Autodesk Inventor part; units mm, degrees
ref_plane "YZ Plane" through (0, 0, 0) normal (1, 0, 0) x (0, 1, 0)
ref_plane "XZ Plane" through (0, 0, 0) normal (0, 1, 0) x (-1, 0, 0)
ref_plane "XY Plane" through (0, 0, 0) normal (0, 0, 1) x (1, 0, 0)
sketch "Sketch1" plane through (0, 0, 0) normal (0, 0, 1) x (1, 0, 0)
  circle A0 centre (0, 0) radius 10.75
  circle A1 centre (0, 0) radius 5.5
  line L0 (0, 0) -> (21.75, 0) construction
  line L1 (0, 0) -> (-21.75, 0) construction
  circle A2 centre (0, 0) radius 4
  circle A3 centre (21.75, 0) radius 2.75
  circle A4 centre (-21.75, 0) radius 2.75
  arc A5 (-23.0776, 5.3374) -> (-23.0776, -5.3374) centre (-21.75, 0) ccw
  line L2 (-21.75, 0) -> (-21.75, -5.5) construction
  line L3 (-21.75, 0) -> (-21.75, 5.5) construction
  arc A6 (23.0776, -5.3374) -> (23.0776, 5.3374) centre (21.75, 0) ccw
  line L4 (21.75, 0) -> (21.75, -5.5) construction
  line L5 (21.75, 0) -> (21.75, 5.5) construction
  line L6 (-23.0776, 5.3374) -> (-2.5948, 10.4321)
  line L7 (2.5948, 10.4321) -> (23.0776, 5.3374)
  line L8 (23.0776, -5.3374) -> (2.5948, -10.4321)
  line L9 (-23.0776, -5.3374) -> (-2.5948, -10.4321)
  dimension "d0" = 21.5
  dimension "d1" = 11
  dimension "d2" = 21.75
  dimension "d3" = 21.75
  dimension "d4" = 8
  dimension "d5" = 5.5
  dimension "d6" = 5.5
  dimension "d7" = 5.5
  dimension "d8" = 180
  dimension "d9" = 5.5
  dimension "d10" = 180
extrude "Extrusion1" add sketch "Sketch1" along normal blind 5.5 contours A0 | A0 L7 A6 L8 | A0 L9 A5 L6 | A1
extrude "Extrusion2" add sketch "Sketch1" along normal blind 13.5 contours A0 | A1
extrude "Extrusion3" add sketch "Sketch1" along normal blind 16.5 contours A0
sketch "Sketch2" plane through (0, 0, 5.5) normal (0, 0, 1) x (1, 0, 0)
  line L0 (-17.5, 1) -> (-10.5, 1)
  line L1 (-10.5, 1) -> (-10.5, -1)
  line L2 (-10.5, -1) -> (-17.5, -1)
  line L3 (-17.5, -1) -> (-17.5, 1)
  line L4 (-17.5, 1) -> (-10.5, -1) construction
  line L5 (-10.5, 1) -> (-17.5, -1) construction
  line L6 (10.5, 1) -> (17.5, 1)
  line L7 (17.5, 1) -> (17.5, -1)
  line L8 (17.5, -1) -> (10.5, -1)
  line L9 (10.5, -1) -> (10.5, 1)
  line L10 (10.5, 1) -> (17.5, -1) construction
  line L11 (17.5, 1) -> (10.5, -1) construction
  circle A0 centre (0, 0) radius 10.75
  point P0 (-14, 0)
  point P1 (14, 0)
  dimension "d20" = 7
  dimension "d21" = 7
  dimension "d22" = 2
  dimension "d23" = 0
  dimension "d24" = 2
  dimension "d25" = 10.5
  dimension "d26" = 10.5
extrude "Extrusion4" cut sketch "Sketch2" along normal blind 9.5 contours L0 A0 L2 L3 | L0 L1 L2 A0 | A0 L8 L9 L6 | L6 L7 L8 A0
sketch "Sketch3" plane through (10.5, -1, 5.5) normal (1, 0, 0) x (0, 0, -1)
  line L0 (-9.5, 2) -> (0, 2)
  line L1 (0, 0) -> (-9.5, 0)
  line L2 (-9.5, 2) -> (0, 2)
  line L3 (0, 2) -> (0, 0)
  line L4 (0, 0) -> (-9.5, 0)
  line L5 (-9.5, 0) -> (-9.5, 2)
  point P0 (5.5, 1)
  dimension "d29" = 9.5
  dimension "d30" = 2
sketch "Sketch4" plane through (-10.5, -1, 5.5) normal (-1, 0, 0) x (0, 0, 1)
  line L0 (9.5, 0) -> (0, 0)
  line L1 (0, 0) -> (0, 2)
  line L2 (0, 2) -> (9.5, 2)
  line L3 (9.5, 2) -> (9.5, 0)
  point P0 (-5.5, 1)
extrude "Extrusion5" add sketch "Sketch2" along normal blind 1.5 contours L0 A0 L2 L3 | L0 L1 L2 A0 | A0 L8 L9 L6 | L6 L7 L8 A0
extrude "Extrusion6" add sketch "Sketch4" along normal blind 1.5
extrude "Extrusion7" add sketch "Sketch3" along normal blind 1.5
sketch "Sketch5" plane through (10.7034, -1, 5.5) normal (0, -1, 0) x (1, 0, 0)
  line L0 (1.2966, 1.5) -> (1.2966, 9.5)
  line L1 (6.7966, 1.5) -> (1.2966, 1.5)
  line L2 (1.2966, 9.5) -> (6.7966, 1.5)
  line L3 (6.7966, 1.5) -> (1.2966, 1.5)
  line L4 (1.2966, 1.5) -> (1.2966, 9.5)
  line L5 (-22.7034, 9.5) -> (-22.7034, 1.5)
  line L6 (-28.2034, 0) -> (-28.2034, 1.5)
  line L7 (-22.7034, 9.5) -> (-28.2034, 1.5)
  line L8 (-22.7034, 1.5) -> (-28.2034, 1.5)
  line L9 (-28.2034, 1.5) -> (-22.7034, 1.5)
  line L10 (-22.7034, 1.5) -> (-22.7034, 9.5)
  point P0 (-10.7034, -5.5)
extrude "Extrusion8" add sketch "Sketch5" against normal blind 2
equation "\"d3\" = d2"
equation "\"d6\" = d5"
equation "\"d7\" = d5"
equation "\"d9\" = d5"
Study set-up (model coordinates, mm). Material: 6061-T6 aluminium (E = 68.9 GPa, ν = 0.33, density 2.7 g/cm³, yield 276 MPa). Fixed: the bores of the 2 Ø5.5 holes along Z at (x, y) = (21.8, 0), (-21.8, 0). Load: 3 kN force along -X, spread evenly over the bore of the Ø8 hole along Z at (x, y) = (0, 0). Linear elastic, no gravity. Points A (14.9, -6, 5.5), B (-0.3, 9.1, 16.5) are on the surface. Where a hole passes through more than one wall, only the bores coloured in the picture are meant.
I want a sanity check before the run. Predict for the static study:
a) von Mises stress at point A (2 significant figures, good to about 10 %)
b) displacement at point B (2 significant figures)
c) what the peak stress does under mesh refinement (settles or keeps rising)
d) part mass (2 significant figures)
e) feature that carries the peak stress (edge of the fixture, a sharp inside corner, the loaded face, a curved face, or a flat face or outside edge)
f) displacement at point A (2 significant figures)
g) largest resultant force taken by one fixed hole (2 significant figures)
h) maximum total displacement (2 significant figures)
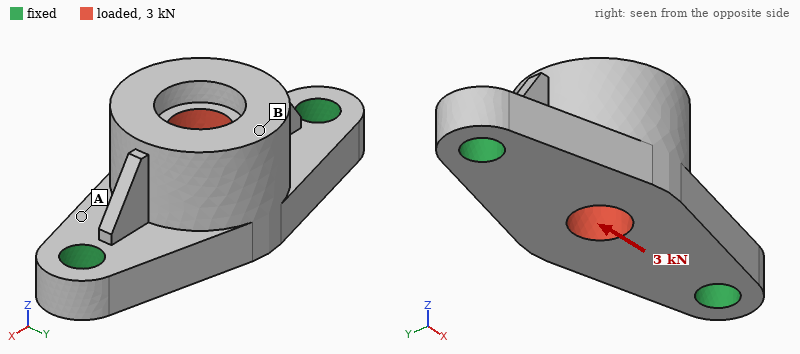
18 MPa
6.5 µm
keeps rising
20 g
a sharp inside corner
2.3 µm
1.5 kN
6.8 µm
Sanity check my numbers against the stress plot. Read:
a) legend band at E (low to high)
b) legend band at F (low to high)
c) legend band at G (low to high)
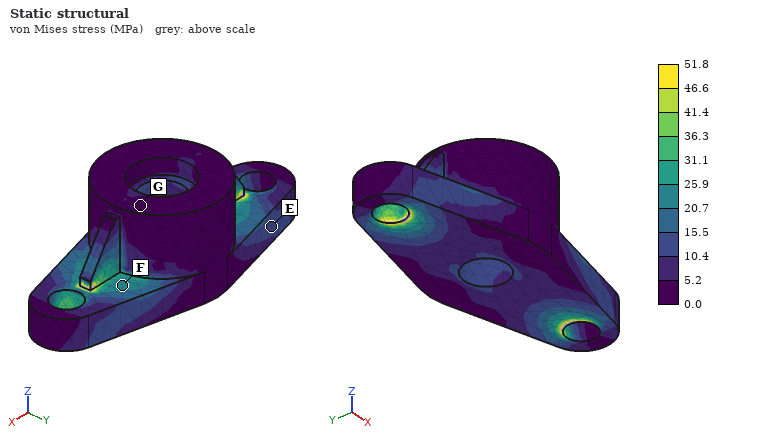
10.4 to 15.5 MPa
20.7 to 25.9 MPa
0.0 to 5.2 MPa
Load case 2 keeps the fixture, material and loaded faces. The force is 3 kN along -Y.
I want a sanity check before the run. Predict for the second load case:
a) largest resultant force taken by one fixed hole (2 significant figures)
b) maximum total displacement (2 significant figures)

1.5 kN
77 µm
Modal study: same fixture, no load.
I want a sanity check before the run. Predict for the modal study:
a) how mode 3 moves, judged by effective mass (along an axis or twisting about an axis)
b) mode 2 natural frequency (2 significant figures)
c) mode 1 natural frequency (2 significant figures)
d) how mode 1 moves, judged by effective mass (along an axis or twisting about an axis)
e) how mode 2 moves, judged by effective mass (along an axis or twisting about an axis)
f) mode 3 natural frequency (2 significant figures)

along Y
14 kHz
8000 Hz
along Y
along Z
21 kHz
